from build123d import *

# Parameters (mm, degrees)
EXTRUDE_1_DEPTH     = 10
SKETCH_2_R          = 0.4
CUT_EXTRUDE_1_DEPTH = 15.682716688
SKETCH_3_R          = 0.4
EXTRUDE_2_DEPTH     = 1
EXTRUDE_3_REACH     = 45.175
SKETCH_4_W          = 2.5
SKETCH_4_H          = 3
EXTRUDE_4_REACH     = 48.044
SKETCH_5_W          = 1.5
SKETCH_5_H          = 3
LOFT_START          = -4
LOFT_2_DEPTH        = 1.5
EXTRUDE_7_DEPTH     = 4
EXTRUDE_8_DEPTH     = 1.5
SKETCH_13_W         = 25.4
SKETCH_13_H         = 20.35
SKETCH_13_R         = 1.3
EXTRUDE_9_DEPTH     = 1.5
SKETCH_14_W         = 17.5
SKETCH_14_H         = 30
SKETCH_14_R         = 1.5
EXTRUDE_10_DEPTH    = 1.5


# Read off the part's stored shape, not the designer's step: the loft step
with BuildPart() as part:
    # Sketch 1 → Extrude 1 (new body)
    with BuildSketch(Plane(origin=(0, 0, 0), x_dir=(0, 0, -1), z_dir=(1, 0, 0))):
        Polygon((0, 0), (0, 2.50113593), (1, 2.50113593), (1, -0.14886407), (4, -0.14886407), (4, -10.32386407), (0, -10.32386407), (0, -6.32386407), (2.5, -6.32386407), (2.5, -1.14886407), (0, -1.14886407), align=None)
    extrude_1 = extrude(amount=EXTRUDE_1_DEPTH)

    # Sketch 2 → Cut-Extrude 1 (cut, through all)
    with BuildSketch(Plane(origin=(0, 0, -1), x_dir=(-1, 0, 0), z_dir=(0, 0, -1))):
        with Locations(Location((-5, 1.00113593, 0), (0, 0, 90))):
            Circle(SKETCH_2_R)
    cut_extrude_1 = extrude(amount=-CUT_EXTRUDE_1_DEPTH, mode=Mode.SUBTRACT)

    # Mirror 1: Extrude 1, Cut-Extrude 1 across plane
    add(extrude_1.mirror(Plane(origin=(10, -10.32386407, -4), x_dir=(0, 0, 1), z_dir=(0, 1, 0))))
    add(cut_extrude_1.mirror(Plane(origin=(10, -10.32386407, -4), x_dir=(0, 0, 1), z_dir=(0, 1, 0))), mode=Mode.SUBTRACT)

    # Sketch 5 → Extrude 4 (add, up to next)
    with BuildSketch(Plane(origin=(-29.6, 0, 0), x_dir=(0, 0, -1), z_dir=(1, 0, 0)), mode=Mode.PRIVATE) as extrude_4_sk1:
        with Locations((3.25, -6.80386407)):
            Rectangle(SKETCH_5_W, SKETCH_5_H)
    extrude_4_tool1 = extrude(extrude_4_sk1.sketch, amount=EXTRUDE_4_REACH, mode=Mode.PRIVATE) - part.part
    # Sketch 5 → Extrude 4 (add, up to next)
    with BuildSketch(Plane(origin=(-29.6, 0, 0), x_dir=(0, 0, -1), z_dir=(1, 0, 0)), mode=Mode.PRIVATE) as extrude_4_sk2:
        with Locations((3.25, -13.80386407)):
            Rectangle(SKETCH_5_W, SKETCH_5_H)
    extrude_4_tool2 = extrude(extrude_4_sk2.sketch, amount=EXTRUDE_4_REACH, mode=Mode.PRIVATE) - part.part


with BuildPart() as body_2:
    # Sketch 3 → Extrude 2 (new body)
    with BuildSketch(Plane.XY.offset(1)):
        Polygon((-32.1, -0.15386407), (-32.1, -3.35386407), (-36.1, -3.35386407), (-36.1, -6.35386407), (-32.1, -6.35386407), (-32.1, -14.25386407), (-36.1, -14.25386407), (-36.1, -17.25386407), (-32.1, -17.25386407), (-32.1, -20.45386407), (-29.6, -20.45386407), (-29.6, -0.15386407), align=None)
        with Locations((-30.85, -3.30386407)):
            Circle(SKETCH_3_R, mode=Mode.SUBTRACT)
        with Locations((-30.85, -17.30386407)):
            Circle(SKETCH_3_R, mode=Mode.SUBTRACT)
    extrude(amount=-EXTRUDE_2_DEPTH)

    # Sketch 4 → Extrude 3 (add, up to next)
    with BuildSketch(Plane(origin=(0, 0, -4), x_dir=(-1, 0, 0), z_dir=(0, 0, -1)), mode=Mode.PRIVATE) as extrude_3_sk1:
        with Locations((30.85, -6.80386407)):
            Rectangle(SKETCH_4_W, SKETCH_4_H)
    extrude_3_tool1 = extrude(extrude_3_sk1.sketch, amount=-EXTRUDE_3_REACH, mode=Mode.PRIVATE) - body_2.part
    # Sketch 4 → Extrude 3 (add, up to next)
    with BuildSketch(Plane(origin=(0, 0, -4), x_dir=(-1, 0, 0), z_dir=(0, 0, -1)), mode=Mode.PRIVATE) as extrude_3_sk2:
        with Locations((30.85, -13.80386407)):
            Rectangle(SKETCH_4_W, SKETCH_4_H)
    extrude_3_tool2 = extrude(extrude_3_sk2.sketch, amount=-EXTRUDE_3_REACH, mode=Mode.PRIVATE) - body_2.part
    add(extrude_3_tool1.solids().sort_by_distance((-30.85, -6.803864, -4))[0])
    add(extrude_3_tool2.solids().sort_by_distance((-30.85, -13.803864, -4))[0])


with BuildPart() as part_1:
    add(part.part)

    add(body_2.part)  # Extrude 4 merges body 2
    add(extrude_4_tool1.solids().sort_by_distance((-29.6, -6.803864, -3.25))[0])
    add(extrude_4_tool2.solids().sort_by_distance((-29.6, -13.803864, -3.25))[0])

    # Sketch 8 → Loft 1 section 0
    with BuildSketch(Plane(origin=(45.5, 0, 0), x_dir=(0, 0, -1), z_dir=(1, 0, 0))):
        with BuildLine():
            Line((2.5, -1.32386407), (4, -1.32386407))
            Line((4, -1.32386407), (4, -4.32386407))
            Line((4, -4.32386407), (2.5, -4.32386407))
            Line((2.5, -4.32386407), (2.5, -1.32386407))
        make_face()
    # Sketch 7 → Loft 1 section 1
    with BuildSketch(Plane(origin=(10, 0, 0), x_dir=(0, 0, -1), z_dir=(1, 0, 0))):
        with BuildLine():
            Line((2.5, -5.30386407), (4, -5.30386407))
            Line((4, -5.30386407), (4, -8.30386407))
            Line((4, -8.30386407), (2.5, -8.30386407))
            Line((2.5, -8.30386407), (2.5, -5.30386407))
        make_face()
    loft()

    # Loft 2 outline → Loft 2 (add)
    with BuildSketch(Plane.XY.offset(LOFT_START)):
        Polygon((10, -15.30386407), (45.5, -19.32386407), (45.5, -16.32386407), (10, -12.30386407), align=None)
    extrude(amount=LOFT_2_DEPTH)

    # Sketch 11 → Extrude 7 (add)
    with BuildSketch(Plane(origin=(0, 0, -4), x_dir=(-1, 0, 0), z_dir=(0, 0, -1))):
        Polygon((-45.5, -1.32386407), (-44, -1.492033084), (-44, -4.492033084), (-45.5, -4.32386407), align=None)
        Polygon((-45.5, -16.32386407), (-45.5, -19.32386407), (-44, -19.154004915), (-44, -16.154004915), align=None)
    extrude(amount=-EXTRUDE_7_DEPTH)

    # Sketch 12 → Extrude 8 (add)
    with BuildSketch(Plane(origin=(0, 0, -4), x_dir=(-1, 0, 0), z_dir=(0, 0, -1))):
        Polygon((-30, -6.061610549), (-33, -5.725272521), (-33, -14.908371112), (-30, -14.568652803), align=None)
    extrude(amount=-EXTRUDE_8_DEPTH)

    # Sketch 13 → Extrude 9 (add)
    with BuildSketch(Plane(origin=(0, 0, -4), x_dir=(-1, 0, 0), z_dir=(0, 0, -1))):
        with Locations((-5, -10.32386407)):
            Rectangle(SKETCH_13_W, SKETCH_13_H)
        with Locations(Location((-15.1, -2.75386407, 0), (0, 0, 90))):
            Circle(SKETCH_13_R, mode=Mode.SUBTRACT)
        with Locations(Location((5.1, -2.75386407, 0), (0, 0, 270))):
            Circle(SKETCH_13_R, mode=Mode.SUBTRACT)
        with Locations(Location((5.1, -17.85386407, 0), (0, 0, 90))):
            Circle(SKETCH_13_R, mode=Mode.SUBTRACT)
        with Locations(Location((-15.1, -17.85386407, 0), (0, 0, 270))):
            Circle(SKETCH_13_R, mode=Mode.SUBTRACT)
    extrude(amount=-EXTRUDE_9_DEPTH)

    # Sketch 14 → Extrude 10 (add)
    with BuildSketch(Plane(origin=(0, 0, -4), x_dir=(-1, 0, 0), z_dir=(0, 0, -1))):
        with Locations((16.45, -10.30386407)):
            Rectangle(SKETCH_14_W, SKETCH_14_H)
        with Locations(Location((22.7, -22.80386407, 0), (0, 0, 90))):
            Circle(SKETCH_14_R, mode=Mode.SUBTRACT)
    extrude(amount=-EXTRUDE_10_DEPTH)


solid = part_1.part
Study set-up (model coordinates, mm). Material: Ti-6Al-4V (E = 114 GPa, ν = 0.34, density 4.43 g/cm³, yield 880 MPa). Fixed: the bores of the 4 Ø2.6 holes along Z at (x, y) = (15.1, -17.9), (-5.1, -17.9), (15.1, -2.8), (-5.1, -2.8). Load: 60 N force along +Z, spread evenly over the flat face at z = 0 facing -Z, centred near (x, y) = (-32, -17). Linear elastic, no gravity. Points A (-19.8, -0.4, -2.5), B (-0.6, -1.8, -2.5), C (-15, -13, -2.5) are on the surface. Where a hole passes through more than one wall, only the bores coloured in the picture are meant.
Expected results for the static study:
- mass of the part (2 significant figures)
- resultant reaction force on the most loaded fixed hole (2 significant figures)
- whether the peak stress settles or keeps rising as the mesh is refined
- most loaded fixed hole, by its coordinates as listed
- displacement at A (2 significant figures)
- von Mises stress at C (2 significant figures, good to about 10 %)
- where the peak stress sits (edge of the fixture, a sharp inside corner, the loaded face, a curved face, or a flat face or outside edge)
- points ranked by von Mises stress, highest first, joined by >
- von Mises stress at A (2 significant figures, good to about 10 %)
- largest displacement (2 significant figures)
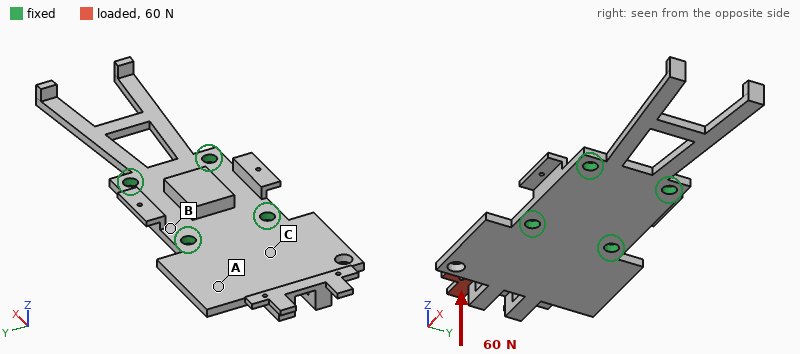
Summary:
10 g
60 N
keeps rising
(-5.1, -17.9)
0.14 mm
110 MPa
edge of the fixture
C > A > B
62 MPa
0.83 mm
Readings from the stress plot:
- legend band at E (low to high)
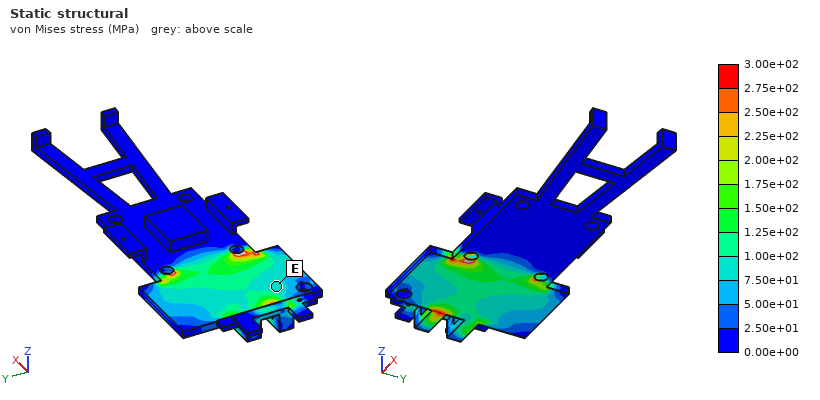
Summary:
7.50e+01 to 1.00e+02 MPa
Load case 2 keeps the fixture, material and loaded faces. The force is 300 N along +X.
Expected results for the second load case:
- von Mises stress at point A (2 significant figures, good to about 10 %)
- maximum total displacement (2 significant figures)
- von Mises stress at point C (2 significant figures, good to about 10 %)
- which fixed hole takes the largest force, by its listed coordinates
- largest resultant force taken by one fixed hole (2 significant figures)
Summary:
65 MPa
0.95 mm
110 MPa
(-5.1, -17.9)
260 N
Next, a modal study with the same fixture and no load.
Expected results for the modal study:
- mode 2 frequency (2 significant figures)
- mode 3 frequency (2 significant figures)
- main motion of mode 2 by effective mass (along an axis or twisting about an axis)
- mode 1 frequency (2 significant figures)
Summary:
1700 Hz
2500 Hz
along Z
1200 Hz
